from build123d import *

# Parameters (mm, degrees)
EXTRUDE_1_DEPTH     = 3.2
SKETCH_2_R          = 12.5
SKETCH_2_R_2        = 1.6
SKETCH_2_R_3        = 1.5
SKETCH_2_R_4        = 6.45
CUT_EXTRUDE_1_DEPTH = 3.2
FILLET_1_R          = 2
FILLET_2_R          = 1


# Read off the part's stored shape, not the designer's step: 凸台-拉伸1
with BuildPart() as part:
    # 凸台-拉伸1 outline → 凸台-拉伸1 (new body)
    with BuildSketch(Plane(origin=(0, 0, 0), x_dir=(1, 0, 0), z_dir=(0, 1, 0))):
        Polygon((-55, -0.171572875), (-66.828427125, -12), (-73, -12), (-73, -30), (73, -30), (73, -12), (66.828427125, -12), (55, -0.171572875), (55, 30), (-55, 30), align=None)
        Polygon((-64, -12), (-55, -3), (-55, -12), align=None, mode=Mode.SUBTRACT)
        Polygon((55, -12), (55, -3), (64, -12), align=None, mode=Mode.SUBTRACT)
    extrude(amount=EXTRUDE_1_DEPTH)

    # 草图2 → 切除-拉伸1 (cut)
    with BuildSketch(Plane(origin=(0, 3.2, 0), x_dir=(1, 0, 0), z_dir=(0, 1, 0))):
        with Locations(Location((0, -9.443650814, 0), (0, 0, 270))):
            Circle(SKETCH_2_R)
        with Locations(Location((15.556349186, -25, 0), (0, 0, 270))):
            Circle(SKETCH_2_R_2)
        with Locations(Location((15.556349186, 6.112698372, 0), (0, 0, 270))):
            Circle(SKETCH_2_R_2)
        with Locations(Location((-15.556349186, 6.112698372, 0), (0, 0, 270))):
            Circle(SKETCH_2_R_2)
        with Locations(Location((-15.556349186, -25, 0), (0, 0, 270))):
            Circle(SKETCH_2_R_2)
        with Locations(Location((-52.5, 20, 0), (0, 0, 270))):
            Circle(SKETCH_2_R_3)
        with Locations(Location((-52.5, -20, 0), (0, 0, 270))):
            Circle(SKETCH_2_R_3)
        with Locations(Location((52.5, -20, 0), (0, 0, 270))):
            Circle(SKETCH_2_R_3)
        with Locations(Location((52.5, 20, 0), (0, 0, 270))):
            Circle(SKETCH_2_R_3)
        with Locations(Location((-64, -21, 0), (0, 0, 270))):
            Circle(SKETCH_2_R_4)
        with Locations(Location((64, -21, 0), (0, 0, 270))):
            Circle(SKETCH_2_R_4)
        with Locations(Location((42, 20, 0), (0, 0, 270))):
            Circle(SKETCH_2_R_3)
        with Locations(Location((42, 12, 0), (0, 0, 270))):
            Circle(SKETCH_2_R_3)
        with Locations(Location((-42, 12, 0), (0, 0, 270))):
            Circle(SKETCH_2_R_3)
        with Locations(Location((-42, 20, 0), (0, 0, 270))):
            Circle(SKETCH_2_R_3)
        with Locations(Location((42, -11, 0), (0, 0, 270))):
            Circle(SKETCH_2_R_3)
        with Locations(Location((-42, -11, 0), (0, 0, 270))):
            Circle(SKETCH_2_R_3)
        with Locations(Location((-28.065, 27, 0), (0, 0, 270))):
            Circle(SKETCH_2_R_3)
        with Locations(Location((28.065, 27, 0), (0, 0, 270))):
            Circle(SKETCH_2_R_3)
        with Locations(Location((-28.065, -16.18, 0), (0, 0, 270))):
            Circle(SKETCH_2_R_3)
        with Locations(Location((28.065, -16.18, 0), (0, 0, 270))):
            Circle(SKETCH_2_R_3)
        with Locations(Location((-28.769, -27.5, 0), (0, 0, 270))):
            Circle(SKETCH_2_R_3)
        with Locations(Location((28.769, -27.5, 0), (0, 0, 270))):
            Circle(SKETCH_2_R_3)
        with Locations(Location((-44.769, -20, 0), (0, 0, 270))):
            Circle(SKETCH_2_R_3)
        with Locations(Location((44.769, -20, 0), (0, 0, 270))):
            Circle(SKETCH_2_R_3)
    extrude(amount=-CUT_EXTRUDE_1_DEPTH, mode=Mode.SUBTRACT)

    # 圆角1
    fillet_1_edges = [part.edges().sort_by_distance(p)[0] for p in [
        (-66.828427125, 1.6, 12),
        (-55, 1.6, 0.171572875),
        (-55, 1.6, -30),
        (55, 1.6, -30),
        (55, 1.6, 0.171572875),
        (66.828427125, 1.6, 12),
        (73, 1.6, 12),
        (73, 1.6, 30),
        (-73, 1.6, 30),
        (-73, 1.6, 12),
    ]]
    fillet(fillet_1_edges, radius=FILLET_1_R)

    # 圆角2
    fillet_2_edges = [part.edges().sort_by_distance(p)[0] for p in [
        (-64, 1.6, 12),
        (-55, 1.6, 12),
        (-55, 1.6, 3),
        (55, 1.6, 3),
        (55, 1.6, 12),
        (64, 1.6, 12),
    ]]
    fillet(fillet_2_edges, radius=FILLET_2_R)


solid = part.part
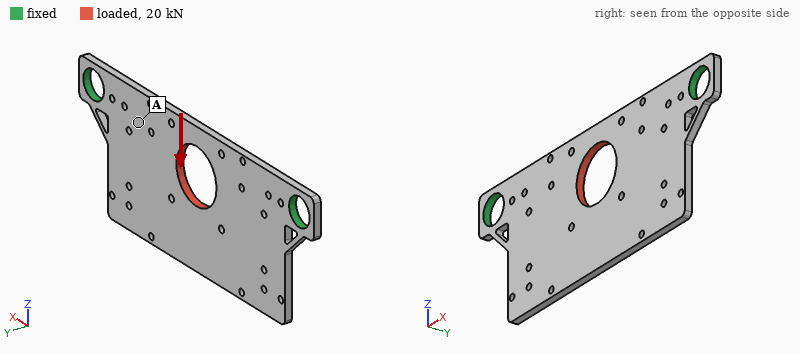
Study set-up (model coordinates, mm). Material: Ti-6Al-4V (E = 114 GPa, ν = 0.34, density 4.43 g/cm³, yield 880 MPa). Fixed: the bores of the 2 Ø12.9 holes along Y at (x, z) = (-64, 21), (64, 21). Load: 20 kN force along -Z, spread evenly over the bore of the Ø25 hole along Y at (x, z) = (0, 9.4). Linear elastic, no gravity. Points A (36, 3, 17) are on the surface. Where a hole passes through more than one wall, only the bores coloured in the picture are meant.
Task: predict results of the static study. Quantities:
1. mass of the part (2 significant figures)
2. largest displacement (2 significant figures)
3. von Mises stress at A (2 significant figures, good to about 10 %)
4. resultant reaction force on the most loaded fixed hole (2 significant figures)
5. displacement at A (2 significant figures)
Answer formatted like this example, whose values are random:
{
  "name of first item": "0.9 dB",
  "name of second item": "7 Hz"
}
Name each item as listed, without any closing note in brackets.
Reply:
{
  "mass of the part": "91 g",
  "largest displacement": "0.22 mm",
  "von Mises stress at A": "84 MPa",
  "resultant reaction force on the most loaded fixed hole": "12 kN",
  "displacement at A": "0.11 mm"
}
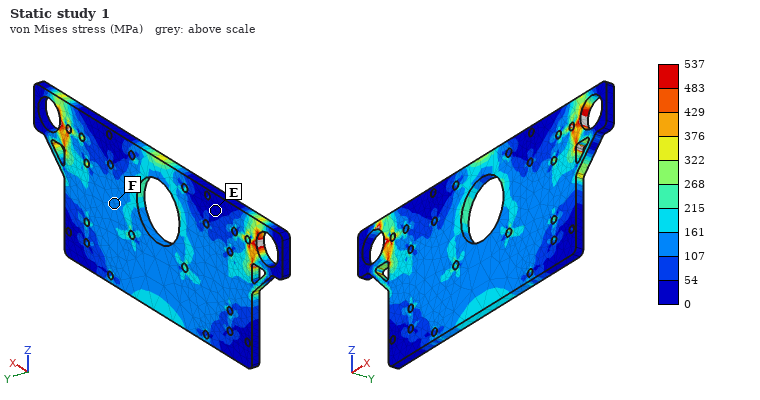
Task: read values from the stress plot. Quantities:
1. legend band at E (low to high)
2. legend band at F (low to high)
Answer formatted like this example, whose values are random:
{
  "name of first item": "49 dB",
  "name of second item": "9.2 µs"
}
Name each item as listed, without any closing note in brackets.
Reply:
{
  "legend band at E": "0 to 54 MPa",
  "legend band at F": "107 to 161 MPa"
}
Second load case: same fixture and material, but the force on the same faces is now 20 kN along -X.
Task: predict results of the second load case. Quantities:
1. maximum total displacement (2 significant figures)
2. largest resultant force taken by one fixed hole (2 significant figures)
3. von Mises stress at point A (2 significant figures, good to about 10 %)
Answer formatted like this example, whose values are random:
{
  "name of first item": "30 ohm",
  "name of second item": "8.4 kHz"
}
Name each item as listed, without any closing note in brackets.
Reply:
{
  "maximum total displacement": "71 µm",
  "largest resultant force taken by one fixed hole": "10 kN",
  "von Mises stress at point A": "100 MPa"
}
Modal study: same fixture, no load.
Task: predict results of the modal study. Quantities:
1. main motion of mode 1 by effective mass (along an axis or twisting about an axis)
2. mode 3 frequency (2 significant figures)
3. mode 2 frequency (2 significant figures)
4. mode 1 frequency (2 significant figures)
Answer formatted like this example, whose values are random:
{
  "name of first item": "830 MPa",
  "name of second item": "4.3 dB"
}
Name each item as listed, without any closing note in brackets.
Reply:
{
  "main motion of mode 1 by effective mass": "along Y",
  "mode 3 frequency": "1400 Hz",
  "mode 2 frequency": "1400 Hz",
  "mode 1 frequency": "560 Hz"
}
